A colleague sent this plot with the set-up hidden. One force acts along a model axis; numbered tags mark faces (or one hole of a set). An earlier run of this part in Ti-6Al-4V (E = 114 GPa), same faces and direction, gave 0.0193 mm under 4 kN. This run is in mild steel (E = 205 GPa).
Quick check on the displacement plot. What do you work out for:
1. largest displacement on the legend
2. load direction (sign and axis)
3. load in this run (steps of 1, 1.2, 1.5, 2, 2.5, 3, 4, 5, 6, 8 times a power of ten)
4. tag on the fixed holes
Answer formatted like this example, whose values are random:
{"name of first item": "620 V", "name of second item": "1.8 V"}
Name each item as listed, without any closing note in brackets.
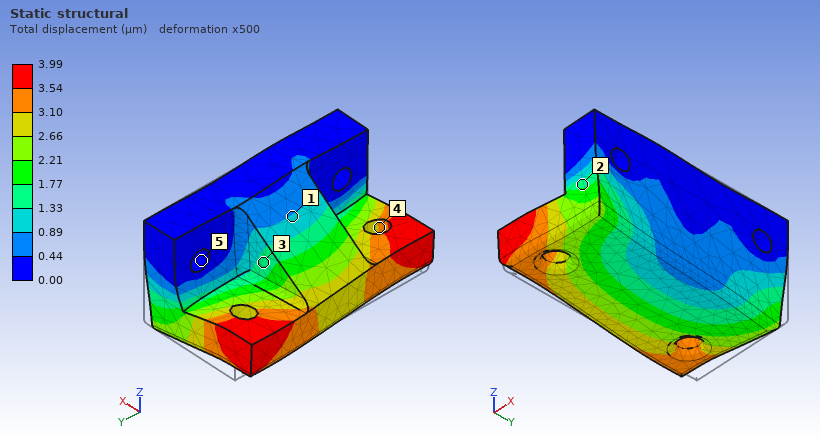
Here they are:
{"largest displacement on the legend": "3.99 µm", "load direction": "-Y", "load in this run": "1.5 kN", "tag on the fixed holes": "5"}
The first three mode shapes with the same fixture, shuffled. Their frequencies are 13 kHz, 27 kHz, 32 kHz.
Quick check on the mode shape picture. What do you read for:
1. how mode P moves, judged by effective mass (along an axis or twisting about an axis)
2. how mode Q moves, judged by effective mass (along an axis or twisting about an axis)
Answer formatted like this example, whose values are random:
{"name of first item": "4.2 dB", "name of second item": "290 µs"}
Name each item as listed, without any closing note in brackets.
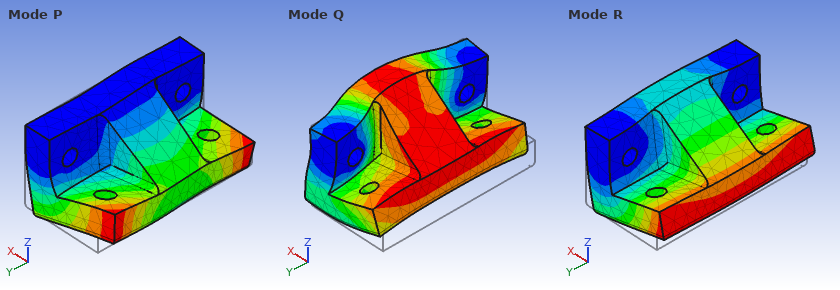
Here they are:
{"how mode P moves, judged by effective mass": "along Y", "how mode Q moves, judged by effective mass": "along X"}
